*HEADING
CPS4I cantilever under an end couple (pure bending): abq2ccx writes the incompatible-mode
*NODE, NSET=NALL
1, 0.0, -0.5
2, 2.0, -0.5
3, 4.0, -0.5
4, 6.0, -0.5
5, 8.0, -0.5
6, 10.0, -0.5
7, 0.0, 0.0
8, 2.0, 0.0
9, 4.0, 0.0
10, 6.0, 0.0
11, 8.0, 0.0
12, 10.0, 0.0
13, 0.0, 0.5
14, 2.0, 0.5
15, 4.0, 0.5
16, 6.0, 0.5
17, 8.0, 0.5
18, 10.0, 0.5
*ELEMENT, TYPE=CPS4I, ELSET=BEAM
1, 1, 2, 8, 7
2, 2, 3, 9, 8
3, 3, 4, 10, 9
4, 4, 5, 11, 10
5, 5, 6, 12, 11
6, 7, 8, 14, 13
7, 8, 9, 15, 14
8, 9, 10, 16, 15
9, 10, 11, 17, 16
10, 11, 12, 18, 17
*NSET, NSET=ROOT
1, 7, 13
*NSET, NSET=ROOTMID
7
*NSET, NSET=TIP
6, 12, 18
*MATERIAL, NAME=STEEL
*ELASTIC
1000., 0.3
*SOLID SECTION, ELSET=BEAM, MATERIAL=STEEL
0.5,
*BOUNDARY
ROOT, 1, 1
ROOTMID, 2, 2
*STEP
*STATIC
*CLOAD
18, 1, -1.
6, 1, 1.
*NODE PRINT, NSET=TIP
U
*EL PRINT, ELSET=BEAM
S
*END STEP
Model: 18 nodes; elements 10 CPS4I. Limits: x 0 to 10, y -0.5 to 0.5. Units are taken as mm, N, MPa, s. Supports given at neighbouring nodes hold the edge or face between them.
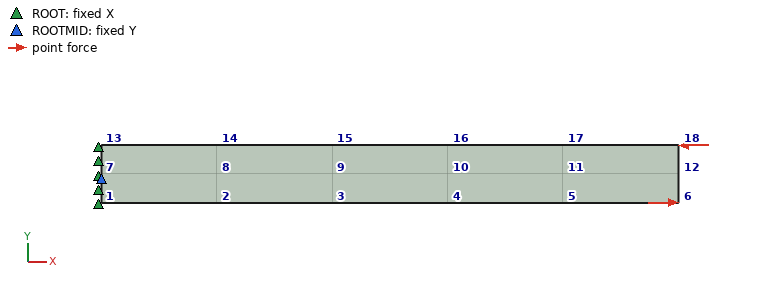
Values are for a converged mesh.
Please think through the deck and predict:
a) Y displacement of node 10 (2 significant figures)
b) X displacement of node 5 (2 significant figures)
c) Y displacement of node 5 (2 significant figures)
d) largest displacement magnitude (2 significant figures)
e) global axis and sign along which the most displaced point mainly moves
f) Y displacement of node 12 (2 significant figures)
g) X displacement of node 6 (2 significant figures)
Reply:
0.43 mm
0.095 mm
0.76 mm
1.2 mm
+Y
1.2 mm
0.12 mm
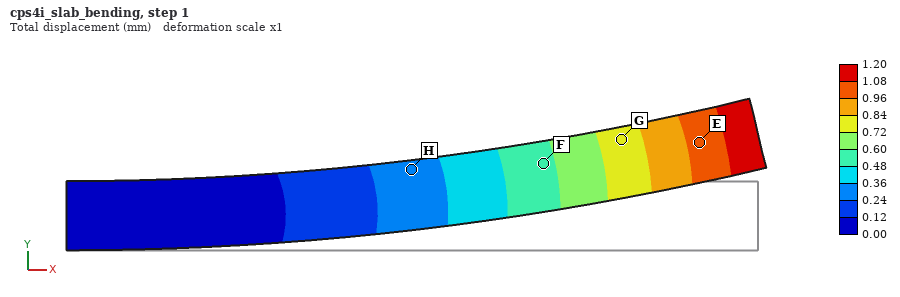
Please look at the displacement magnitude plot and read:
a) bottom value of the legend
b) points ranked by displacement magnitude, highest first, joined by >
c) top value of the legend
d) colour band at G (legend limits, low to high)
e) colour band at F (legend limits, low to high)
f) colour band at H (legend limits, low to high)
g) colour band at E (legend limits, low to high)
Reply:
0.00 mm
E > G > F > H
1.20 mm
0.72 to 0.84 mm
0.48 to 0.60 mm
0.24 to 0.36 mm
0.96 to 1.08 mm
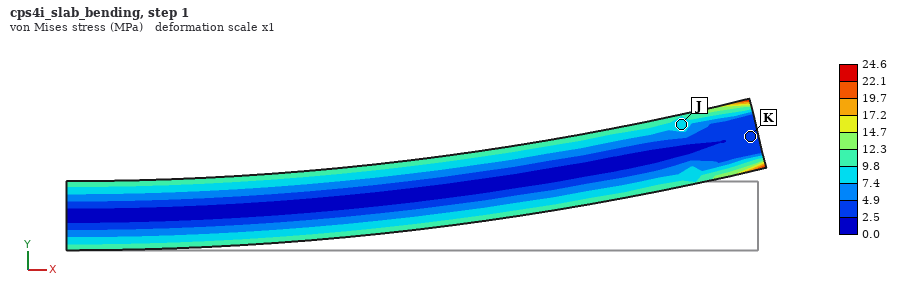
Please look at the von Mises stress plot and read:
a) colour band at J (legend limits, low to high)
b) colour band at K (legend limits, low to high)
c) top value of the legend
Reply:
7.4 to 9.8 MPa
2.5 to 4.9 MPa
24.6 MPa
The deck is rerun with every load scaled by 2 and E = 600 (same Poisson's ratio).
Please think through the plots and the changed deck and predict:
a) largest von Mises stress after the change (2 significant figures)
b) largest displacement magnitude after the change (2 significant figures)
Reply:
49 MPa
4.0 mm
